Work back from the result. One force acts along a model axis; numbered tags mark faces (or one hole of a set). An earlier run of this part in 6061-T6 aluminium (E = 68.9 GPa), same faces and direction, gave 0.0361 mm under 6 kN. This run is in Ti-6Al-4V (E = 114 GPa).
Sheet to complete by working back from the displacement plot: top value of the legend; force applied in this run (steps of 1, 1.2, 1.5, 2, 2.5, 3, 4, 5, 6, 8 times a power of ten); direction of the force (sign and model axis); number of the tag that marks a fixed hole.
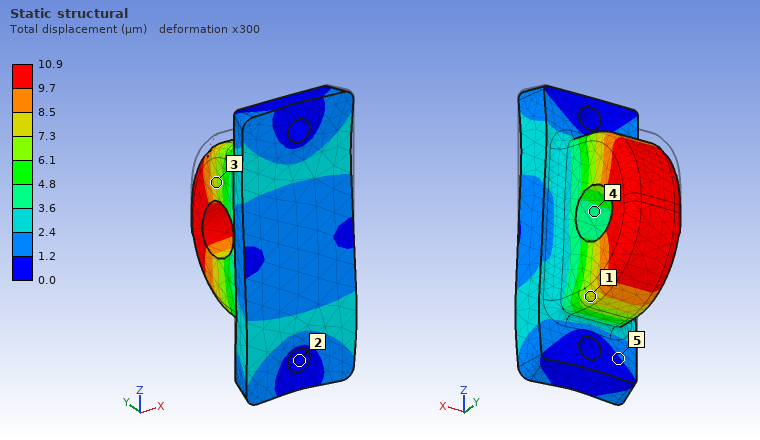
10.9 µm
3 kN
-Z
2
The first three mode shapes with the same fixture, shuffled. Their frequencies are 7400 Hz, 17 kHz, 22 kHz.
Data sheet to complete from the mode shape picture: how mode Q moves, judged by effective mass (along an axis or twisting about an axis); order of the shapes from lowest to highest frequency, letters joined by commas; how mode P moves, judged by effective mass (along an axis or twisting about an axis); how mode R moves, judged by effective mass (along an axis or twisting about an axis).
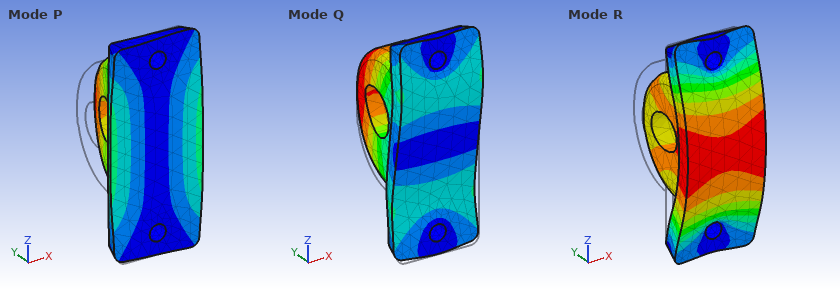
along Z
P, R, Q
along X
along Y
